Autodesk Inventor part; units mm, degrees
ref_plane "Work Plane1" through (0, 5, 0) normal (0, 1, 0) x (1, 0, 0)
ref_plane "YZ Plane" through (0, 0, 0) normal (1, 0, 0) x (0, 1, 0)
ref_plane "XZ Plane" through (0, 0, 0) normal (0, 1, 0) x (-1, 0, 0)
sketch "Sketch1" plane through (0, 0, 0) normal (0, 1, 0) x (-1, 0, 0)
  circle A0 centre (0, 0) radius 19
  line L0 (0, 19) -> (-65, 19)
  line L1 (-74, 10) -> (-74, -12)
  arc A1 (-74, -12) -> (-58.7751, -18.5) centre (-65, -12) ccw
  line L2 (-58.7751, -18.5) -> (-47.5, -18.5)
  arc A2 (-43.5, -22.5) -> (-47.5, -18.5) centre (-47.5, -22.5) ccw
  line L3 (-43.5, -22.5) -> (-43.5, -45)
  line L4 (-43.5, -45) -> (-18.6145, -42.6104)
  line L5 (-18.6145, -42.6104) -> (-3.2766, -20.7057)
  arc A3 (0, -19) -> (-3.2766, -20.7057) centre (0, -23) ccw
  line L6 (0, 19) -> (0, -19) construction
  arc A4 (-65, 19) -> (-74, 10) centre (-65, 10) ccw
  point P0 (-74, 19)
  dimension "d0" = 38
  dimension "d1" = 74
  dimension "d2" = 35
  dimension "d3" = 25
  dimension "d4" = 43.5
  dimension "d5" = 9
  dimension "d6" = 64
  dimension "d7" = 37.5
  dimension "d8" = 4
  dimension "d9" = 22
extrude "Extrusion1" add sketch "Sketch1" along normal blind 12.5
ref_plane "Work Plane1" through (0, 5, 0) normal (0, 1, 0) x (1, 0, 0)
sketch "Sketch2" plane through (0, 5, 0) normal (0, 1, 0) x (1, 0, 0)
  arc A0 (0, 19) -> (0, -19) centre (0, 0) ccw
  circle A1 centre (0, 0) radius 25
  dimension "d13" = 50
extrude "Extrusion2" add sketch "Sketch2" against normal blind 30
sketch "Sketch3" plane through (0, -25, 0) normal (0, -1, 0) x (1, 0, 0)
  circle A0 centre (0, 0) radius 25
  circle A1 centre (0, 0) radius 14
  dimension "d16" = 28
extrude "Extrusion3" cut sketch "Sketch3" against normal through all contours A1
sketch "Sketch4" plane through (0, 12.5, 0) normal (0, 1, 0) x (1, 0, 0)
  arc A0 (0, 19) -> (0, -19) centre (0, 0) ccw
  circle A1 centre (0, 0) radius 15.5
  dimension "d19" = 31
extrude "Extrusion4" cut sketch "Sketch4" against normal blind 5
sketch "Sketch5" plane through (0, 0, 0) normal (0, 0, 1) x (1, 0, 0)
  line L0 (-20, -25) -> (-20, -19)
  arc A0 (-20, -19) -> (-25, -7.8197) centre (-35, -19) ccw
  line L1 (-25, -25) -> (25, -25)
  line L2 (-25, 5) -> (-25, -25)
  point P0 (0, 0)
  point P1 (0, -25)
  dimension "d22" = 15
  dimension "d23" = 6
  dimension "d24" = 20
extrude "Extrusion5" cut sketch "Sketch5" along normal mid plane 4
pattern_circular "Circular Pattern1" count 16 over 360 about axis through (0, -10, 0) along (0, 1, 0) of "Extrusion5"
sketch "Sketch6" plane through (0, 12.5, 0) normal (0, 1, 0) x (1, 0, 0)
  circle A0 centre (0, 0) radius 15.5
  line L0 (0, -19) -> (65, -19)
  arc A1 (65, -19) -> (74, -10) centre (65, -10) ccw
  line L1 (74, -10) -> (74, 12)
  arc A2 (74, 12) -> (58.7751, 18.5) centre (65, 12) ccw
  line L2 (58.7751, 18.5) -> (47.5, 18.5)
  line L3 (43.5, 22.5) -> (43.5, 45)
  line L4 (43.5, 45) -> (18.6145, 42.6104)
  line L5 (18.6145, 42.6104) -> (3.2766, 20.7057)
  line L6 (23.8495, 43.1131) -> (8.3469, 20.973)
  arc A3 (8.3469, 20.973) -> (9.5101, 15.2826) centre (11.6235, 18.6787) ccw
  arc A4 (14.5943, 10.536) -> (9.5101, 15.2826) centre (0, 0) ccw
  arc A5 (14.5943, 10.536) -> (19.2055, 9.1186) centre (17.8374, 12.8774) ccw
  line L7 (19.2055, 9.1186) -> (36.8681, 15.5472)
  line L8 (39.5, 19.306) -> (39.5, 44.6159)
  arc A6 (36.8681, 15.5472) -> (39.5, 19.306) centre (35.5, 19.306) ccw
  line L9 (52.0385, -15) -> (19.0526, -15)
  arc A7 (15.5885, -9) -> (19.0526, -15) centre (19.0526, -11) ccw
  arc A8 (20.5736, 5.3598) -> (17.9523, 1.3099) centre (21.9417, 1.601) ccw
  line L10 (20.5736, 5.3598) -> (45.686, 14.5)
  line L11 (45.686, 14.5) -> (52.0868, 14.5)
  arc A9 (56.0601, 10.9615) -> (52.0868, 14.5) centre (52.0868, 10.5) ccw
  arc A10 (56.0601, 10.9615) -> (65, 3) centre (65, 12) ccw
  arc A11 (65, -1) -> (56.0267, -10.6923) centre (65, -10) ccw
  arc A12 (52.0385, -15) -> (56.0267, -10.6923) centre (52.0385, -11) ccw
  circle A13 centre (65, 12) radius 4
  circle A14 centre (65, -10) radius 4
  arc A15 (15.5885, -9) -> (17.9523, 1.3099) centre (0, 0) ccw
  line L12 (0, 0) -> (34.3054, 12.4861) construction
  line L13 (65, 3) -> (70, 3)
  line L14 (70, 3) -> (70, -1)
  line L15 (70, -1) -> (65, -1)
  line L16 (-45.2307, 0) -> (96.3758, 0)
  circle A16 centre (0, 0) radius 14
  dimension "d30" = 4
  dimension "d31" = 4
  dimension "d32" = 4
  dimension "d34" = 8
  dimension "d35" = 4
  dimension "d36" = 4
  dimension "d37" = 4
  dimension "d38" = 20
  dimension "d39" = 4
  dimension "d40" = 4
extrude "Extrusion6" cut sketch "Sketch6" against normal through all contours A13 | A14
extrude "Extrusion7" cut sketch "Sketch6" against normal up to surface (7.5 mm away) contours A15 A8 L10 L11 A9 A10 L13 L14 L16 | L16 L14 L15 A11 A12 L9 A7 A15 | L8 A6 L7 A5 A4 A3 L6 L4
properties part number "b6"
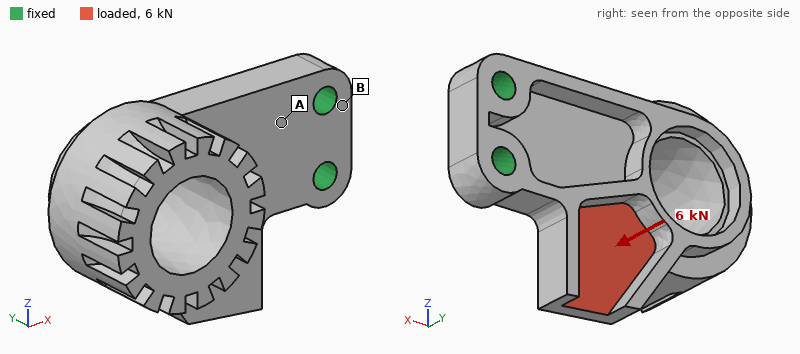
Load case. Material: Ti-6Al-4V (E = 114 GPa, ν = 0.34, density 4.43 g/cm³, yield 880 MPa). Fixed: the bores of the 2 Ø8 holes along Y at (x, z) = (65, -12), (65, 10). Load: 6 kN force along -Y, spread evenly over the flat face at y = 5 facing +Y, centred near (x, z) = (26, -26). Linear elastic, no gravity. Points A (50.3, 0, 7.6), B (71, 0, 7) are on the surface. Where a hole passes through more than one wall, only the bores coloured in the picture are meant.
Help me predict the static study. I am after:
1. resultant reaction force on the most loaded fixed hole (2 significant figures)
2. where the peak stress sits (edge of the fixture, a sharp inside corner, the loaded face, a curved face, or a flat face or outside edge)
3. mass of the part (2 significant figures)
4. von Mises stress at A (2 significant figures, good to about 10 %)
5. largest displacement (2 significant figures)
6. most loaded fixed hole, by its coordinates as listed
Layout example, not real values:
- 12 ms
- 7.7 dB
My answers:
- 8.0 kN
- a curved face
- 270 g
- 180 MPa
- 1.3 mm
- (65, -12)
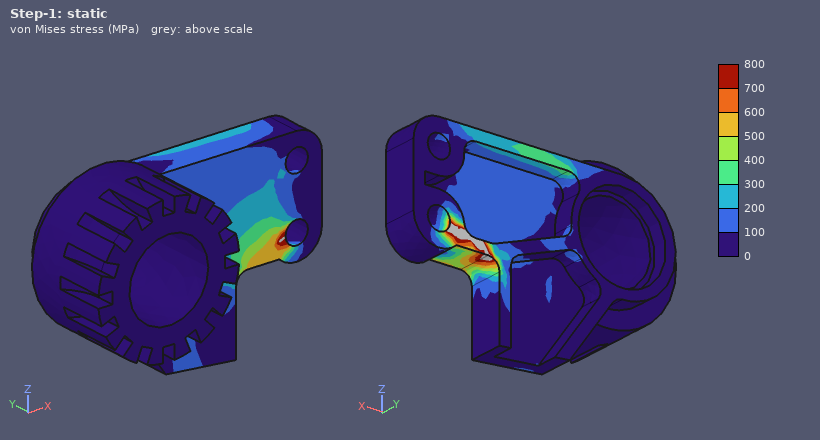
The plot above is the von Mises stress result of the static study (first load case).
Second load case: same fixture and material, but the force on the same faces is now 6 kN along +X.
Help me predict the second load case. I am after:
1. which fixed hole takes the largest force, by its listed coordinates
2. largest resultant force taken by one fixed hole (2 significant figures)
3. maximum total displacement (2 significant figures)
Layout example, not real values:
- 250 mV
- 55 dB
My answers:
- (65, -12)
- 8.6 kN
- 0.12 mm
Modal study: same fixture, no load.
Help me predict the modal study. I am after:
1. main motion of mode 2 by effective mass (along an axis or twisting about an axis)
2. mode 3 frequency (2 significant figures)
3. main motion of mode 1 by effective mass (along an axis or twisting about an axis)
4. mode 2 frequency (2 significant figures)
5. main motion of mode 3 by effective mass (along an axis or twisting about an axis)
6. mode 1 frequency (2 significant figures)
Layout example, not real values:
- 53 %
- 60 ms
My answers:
- along Z
- 2200 Hz
- along Y
- 1600 Hz
- along Z
- 640 Hz
